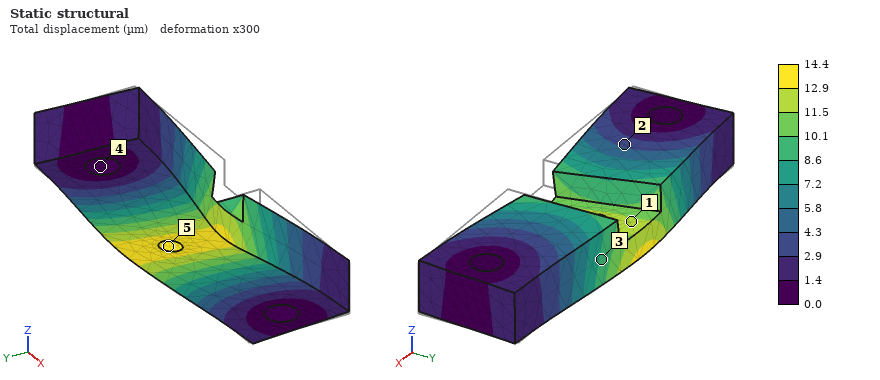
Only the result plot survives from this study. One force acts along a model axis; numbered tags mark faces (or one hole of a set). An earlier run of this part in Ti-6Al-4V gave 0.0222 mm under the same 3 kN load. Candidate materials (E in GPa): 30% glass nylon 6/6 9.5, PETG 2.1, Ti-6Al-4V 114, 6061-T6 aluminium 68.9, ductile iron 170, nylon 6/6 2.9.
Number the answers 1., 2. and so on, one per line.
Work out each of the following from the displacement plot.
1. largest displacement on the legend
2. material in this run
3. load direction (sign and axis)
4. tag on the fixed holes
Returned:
1. 14.4 µm
2. ductile iron
3. +Y
4. 4
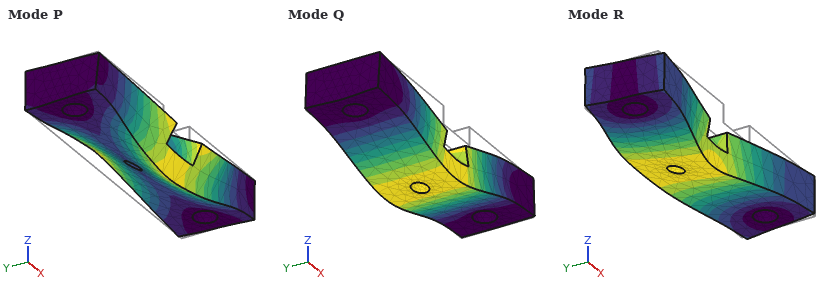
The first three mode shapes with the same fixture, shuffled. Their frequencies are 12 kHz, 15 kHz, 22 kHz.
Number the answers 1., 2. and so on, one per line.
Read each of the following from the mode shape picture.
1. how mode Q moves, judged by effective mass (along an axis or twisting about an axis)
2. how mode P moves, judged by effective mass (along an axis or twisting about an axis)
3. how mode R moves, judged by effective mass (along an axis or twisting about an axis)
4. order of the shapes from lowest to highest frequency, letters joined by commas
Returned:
1. along Z
2. twisting about X
3. along Y
4. Q, R, P
